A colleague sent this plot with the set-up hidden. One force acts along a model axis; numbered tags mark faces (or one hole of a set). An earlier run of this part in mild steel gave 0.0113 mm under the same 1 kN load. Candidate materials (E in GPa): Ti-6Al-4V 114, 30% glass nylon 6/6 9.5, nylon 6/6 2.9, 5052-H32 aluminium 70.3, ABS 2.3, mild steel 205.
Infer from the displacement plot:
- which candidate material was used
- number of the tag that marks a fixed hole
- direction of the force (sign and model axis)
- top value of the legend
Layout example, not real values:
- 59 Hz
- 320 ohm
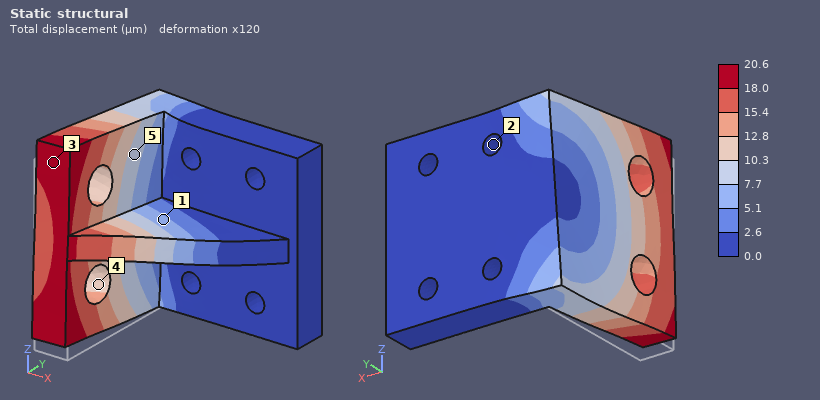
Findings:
- Ti-6Al-4V
- 2
- +Z
- 20.6 µm
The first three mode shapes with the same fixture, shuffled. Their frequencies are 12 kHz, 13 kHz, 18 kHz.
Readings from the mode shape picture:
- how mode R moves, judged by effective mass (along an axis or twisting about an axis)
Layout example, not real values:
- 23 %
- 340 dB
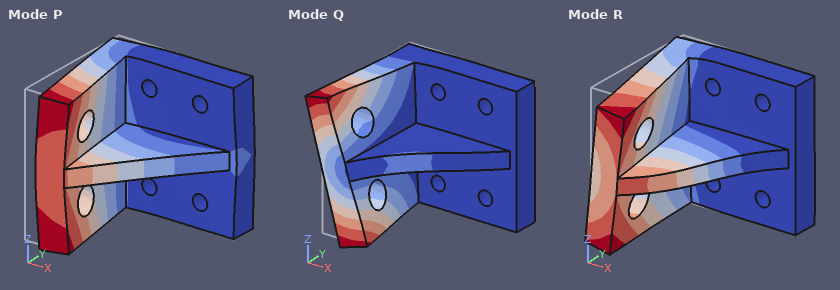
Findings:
- along Z
